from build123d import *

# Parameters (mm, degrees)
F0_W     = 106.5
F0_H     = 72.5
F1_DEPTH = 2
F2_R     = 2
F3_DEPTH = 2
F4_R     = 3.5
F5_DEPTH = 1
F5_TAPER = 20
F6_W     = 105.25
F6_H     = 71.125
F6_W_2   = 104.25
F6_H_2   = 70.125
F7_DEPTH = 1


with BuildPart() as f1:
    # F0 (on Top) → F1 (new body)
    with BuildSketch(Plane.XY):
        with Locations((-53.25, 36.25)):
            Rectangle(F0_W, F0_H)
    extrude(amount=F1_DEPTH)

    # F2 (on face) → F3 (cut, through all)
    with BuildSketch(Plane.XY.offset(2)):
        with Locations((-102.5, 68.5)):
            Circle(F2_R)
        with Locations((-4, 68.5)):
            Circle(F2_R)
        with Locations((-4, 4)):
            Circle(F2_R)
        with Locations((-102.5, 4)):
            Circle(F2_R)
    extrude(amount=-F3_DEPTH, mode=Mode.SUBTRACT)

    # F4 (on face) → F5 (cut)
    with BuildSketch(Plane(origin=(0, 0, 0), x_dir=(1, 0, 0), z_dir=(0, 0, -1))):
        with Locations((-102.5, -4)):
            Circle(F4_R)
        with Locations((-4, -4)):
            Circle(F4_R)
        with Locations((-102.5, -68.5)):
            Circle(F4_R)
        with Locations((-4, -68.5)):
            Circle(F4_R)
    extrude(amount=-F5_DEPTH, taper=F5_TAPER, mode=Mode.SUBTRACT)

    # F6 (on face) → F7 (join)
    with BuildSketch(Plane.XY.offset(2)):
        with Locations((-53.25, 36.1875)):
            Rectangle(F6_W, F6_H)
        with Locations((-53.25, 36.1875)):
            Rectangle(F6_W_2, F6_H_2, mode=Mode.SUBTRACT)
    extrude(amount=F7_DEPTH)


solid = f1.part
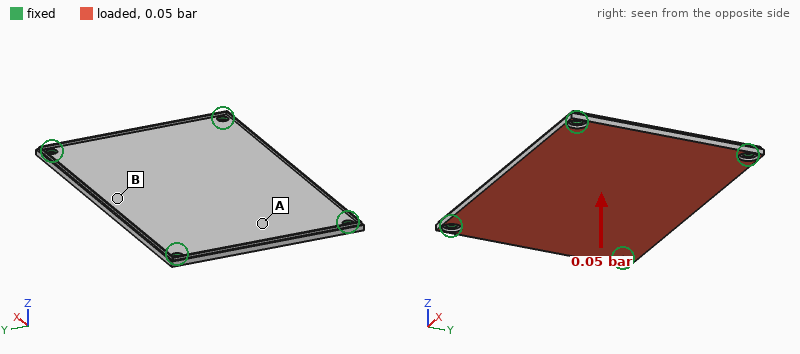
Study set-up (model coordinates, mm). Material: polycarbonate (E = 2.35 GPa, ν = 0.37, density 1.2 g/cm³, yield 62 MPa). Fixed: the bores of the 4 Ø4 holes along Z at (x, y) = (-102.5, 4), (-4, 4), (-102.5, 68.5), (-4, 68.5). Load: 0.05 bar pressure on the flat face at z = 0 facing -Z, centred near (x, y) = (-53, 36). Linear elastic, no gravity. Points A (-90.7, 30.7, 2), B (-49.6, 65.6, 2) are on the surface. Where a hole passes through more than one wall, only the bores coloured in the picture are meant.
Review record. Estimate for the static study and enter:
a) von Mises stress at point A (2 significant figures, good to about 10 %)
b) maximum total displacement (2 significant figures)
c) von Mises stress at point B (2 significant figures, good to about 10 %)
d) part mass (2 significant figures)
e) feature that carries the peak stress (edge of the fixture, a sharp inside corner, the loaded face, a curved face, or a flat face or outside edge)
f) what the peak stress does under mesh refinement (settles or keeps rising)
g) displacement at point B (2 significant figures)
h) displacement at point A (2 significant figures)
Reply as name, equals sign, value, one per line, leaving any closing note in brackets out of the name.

von Mises stress at point A = 1.7 MPa
maximum total displacement = 1.4 mm
von Mises stress at point B = 3.7 MPa
part mass = 19 g
feature that carries the peak stress = edge of the fixture
what the peak stress does under mesh refinement = keeps rising
displacement at point B = 1.3 mm
displacement at point A = 0.62 mm
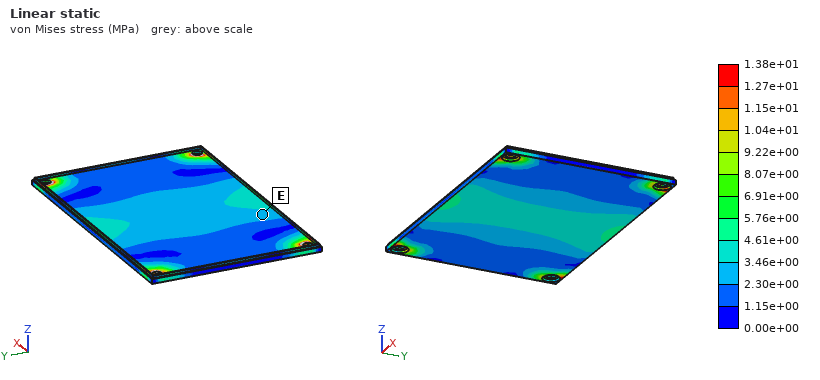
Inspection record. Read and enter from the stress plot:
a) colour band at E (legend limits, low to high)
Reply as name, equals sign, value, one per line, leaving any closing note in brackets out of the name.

colour band at E = 2.30e+00 to 3.46e+00 MPa
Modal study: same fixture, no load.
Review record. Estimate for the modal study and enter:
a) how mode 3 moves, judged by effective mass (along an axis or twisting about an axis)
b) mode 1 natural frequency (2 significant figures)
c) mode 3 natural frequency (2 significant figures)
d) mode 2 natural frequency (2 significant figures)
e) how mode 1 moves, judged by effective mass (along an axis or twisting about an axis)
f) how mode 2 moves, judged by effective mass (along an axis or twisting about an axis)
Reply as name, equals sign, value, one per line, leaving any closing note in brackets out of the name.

how mode 3 moves, judged by effective mass = twisting about Y
mode 1 natural frequency = 220 Hz
mode 3 natural frequency = 560 Hz
mode 2 natural frequency = 380 Hz
how mode 1 moves, judged by effective mass = along Z
how mode 2 moves, judged by effective mass = twisting about X
